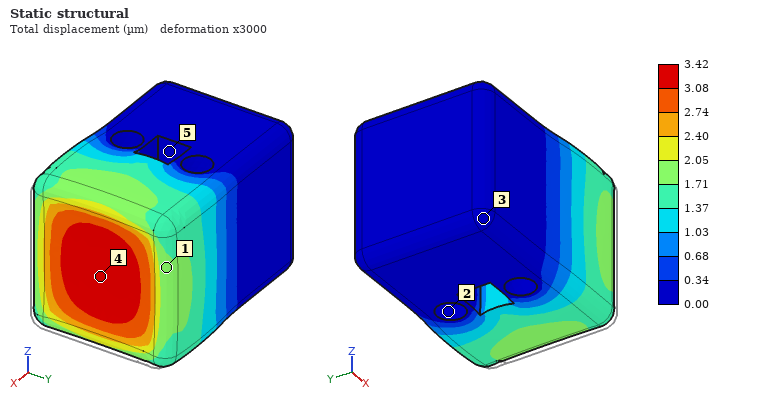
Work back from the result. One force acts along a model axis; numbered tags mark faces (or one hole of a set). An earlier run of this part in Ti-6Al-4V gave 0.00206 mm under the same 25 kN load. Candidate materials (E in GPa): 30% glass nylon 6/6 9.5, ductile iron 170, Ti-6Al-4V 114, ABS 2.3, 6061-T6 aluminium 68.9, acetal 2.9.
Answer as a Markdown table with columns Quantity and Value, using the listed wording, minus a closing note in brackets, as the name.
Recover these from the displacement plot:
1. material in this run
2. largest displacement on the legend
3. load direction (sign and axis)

| Quantity | Value |
|---|---|
| material in this run | 6061-T6 aluminium |
| largest displacement on the legend | 3.42 µm |
| load direction | -X |
